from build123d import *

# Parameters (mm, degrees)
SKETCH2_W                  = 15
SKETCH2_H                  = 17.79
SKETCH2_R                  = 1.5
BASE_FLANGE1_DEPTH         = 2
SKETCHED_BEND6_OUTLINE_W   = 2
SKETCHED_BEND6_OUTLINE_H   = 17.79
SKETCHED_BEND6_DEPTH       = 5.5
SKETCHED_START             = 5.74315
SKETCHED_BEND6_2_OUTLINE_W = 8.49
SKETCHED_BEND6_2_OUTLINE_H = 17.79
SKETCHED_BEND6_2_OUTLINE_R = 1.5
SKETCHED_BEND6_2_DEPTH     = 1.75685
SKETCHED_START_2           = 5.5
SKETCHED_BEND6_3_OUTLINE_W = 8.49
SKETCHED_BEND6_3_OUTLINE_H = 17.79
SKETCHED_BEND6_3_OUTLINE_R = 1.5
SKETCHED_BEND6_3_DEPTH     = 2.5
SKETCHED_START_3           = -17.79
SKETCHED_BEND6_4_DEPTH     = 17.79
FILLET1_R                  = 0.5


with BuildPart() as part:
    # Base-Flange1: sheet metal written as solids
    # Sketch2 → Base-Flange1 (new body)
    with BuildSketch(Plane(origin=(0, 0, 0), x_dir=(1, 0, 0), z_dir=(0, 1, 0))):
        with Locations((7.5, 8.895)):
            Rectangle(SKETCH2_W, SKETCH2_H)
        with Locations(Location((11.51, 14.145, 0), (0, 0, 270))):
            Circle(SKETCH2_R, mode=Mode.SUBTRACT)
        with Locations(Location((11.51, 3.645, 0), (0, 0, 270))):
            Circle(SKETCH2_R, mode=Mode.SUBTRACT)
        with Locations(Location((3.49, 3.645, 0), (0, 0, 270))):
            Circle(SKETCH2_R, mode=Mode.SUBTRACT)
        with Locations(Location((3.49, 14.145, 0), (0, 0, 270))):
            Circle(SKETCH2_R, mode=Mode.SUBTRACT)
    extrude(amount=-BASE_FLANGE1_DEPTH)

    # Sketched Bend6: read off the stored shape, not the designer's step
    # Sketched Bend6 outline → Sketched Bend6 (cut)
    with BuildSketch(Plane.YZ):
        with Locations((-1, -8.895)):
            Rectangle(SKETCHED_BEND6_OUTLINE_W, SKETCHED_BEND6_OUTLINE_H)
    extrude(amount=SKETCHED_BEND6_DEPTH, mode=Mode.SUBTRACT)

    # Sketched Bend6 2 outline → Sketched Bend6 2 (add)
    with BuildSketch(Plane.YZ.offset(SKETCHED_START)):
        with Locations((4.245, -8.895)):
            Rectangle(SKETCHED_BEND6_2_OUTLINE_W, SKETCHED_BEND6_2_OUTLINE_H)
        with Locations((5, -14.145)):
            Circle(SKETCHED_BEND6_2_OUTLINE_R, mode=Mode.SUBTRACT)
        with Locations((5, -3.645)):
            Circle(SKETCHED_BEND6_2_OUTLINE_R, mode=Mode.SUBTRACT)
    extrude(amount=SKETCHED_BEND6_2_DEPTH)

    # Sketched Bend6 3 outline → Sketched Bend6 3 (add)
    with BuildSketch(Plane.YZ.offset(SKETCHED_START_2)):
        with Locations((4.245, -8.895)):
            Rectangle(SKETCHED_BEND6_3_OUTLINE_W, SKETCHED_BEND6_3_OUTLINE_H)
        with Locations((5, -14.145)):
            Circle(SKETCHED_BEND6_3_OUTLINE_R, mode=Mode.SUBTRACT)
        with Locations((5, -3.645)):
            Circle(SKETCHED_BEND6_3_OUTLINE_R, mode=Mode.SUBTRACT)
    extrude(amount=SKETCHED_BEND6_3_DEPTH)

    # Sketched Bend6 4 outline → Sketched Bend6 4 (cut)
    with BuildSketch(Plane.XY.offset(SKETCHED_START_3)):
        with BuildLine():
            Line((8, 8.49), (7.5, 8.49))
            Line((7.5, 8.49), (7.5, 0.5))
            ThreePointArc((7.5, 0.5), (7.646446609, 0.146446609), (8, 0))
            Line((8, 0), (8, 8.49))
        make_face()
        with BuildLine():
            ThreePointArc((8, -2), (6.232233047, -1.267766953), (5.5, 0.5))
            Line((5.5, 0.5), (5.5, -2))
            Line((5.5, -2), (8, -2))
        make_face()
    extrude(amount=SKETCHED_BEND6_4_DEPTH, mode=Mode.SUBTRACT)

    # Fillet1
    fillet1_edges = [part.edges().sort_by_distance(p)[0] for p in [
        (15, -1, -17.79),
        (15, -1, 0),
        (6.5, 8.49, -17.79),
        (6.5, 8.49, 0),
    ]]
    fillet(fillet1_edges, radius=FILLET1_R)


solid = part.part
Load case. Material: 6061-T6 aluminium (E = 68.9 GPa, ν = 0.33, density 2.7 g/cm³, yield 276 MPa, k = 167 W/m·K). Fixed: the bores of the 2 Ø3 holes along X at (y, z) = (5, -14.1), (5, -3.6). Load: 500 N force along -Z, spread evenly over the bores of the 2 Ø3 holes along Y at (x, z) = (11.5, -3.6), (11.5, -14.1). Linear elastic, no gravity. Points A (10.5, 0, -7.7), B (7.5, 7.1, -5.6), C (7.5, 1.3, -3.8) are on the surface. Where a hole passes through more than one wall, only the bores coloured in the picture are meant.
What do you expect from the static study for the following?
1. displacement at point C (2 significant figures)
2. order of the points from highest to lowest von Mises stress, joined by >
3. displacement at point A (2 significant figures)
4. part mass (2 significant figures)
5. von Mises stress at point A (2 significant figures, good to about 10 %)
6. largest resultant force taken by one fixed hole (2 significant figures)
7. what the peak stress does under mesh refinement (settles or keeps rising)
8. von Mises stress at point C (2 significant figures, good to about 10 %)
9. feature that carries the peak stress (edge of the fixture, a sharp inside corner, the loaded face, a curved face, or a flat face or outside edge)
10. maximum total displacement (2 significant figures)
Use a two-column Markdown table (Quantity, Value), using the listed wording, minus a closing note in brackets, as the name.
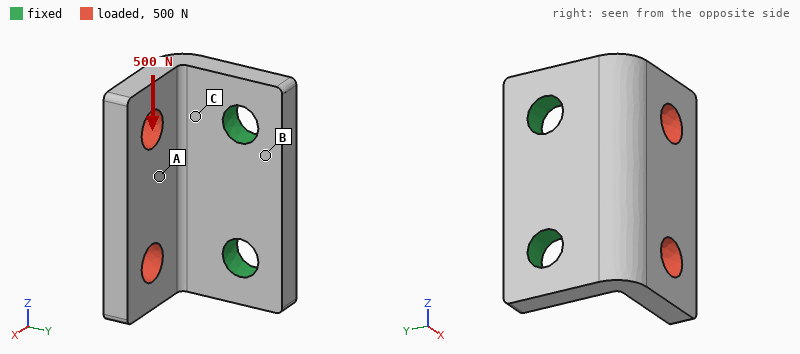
| Quantity | Value |
|---|---|
| displacement at point C | 7.5 µm |
| order of the points from highest to lowest von Mises stress, joined by > | C > A > B |
| displacement at point A | 18 µm |
| part mass | 1.5 g |
| von Mises stress at point A | 52 MPa |
| largest resultant force taken by one fixed hole | 380 N |
| what the peak stress does under mesh refinement | keeps rising |
| von Mises stress at point C | 80 MPa |
| feature that carries the peak stress | edge of the fixture |
| maximum total displacement | 44 µm |
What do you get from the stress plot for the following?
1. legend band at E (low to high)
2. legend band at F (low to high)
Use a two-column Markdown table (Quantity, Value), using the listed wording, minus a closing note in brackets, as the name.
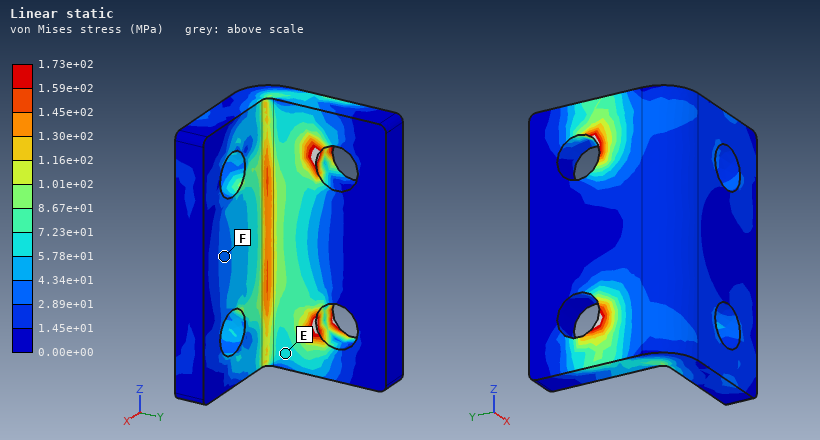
| Quantity | Value |
|---|---|
| legend band at E | 5.78e+01 to 7.23e+01 MPa |
| legend band at F | 2.89e+01 to 4.34e+01 MPa |
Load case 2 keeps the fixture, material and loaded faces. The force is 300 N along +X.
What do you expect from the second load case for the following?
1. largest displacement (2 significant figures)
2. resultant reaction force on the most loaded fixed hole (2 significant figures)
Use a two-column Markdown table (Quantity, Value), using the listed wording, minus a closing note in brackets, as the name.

| Quantity | Value |
|---|---|
| largest displacement | 49 µm |
| resultant reaction force on the most loaded fixed hole | 150 N |
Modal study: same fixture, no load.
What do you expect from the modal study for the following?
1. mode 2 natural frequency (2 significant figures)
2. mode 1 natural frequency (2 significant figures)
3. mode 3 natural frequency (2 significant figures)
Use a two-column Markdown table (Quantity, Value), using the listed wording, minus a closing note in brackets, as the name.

| Quantity | Value |
|---|---|
| mode 2 natural frequency | 20 kHz |
| mode 1 natural frequency | 12 kHz |
| mode 3 natural frequency | 32 kHz |
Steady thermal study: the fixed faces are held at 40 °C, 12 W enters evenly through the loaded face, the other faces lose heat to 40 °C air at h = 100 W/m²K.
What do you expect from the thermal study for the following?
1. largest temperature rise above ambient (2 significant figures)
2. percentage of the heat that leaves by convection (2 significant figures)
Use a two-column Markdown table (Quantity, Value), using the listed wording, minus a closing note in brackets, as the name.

| Quantity | Value |
|---|---|
| largest temperature rise above ambient | 23 K |
| percentage of the heat that leaves by convection | 5.6 % |
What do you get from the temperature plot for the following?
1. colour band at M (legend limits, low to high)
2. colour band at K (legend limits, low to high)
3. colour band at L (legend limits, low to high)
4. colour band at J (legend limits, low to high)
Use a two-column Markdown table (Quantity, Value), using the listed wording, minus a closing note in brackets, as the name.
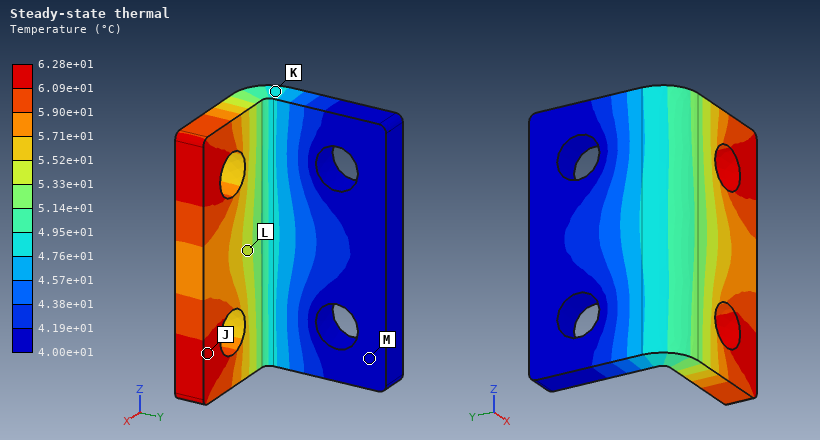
| Quantity | Value |
|---|---|
| colour band at M | 4.00e+01 to 4.19e+01 °C |
| colour band at K | 4.76e+01 to 4.95e+01 °C |
| colour band at L | 5.33e+01 to 5.52e+01 °C |
| colour band at J | 6.09e+01 to 6.28e+01 °C |
